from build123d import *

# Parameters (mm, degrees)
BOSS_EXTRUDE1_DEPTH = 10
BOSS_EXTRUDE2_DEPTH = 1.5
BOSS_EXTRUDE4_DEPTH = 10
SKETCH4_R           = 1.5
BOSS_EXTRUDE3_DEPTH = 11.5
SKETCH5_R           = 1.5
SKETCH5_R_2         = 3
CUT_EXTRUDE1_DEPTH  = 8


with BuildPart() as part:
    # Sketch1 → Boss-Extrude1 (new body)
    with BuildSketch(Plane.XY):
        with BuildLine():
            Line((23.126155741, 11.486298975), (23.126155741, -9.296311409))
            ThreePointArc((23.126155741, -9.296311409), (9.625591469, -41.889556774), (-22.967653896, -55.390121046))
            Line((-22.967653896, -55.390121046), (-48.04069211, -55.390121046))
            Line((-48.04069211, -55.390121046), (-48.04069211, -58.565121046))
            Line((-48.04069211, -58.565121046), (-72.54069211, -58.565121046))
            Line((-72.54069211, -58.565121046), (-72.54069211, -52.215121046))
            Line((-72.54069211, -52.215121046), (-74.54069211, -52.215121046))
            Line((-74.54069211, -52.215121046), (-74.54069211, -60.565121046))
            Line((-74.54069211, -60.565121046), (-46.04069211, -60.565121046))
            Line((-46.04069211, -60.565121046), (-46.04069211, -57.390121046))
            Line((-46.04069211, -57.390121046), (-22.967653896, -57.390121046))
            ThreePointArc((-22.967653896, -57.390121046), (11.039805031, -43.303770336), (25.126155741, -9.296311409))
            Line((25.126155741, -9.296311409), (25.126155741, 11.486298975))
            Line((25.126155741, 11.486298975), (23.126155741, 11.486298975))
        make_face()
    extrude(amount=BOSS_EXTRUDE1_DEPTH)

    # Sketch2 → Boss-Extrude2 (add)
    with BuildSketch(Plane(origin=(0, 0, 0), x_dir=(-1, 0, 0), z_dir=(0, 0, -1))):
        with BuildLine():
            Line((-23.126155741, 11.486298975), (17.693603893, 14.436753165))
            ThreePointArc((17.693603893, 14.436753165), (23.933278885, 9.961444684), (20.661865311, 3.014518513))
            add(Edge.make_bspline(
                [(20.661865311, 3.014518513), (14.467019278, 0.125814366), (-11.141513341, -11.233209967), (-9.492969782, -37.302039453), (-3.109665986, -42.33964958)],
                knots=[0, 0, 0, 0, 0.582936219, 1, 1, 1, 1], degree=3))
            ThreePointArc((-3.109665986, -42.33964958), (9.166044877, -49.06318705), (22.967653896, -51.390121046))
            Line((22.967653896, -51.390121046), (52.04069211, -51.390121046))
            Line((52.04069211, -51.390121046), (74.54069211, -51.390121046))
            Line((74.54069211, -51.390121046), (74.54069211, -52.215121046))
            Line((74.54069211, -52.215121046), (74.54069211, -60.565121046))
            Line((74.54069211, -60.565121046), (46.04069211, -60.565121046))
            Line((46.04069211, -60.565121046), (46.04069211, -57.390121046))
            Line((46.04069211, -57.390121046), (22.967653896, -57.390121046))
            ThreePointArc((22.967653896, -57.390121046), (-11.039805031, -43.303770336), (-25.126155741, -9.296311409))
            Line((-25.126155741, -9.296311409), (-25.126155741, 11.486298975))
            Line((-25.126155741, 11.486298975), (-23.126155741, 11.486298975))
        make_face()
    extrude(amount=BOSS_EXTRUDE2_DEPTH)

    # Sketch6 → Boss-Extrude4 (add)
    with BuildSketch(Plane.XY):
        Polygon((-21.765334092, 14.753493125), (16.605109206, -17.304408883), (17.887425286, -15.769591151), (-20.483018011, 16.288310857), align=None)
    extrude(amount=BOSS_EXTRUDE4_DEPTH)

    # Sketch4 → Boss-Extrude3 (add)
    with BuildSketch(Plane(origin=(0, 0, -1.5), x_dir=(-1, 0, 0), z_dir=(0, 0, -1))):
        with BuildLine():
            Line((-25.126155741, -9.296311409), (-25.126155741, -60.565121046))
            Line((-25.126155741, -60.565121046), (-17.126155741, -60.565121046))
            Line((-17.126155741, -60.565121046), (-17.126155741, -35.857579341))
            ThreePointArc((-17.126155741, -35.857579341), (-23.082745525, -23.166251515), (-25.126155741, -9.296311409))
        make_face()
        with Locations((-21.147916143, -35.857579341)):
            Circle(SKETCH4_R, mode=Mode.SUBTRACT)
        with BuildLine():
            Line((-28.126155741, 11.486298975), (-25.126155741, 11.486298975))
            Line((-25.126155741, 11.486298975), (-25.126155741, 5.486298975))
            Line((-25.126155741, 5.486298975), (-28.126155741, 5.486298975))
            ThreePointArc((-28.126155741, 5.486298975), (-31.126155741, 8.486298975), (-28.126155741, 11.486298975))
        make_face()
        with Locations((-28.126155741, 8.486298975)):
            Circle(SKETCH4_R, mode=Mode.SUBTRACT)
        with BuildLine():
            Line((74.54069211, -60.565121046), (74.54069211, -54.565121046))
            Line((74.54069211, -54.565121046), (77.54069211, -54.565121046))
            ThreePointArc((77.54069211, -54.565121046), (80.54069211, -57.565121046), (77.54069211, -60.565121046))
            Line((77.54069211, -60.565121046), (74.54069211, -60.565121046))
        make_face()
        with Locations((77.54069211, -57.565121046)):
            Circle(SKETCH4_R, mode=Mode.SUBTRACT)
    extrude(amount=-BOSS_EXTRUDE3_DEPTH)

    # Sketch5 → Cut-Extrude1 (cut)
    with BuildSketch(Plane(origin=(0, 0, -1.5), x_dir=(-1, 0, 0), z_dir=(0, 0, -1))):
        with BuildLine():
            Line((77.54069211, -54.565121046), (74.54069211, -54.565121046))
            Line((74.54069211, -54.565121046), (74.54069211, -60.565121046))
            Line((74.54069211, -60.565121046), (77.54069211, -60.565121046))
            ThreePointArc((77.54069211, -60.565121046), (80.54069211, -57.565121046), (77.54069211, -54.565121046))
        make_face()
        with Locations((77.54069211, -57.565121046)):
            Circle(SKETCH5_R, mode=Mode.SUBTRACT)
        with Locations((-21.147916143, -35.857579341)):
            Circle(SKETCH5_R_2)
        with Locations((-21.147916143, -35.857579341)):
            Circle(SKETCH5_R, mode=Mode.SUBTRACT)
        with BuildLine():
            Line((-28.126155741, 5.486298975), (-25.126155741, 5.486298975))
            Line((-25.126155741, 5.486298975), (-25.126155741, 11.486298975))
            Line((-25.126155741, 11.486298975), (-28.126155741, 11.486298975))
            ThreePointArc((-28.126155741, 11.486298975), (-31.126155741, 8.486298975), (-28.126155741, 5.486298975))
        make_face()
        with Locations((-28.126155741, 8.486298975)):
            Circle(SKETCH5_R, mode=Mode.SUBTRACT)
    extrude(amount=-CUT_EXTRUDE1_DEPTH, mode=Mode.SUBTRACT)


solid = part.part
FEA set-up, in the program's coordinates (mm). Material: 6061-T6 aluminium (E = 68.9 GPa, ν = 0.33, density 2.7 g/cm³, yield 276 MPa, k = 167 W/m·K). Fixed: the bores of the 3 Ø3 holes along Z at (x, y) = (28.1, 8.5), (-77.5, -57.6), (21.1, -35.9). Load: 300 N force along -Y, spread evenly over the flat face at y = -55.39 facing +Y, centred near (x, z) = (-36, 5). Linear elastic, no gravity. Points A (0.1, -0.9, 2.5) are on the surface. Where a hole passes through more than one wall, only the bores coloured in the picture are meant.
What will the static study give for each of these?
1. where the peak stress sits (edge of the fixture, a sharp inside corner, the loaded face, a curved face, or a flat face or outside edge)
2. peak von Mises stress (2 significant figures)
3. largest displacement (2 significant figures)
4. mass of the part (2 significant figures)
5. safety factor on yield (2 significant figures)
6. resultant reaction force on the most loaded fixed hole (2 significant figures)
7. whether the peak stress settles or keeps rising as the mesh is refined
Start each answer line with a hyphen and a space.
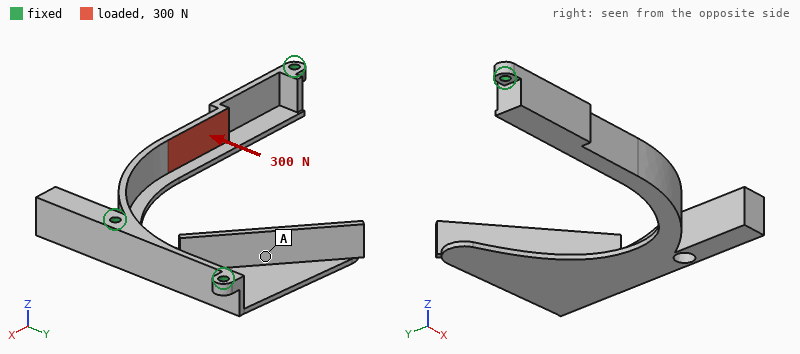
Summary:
- a flat face or outside edge
- 190 MPa
- 0.46 mm
- 27 g
- 1.4
- 350 N
- settles
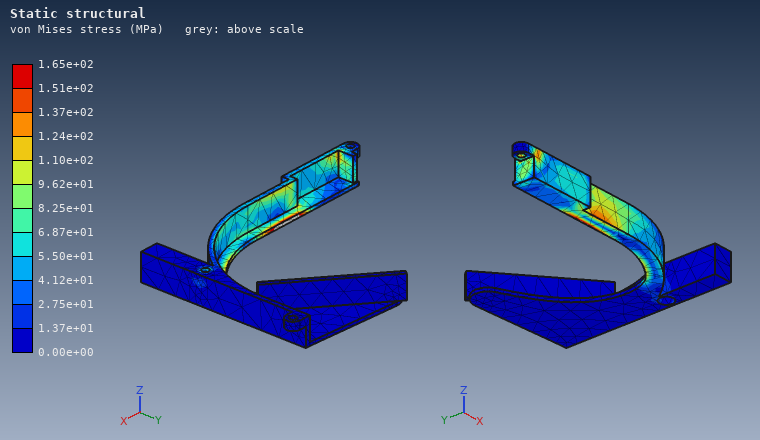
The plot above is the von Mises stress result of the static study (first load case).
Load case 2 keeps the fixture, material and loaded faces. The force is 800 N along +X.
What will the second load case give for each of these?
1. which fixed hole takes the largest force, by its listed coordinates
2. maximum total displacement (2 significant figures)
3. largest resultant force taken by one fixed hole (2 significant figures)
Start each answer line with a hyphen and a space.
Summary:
- (-77.5, -57.6)
- 0.19 mm
- 770 N
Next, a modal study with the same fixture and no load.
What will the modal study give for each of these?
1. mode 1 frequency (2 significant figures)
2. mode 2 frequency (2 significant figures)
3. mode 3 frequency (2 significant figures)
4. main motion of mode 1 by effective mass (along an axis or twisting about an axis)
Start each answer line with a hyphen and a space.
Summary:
- 720 Hz
- 2500 Hz
- 2800 Hz
- along Z
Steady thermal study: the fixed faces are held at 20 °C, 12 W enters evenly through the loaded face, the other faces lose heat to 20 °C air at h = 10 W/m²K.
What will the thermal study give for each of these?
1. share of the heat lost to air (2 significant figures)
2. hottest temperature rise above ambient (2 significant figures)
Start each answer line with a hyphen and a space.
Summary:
- 9.3 %
- 53 K
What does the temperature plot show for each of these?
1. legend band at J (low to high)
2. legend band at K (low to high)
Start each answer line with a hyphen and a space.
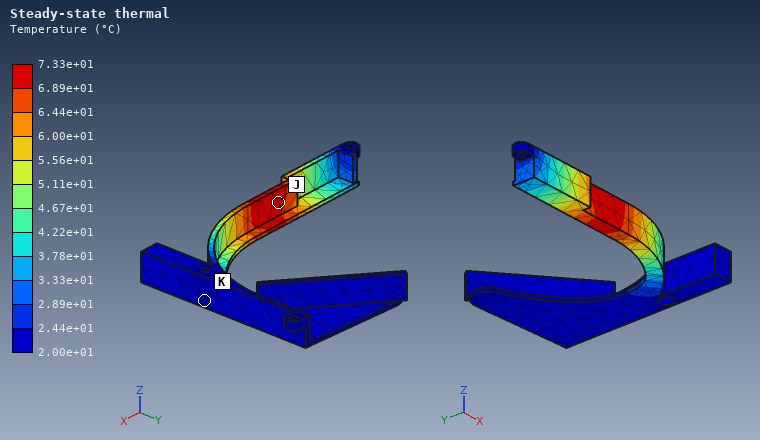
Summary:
- 6.89e+01 to 7.33e+01 °C
- 2.00e+01 to 2.44e+01 °C
